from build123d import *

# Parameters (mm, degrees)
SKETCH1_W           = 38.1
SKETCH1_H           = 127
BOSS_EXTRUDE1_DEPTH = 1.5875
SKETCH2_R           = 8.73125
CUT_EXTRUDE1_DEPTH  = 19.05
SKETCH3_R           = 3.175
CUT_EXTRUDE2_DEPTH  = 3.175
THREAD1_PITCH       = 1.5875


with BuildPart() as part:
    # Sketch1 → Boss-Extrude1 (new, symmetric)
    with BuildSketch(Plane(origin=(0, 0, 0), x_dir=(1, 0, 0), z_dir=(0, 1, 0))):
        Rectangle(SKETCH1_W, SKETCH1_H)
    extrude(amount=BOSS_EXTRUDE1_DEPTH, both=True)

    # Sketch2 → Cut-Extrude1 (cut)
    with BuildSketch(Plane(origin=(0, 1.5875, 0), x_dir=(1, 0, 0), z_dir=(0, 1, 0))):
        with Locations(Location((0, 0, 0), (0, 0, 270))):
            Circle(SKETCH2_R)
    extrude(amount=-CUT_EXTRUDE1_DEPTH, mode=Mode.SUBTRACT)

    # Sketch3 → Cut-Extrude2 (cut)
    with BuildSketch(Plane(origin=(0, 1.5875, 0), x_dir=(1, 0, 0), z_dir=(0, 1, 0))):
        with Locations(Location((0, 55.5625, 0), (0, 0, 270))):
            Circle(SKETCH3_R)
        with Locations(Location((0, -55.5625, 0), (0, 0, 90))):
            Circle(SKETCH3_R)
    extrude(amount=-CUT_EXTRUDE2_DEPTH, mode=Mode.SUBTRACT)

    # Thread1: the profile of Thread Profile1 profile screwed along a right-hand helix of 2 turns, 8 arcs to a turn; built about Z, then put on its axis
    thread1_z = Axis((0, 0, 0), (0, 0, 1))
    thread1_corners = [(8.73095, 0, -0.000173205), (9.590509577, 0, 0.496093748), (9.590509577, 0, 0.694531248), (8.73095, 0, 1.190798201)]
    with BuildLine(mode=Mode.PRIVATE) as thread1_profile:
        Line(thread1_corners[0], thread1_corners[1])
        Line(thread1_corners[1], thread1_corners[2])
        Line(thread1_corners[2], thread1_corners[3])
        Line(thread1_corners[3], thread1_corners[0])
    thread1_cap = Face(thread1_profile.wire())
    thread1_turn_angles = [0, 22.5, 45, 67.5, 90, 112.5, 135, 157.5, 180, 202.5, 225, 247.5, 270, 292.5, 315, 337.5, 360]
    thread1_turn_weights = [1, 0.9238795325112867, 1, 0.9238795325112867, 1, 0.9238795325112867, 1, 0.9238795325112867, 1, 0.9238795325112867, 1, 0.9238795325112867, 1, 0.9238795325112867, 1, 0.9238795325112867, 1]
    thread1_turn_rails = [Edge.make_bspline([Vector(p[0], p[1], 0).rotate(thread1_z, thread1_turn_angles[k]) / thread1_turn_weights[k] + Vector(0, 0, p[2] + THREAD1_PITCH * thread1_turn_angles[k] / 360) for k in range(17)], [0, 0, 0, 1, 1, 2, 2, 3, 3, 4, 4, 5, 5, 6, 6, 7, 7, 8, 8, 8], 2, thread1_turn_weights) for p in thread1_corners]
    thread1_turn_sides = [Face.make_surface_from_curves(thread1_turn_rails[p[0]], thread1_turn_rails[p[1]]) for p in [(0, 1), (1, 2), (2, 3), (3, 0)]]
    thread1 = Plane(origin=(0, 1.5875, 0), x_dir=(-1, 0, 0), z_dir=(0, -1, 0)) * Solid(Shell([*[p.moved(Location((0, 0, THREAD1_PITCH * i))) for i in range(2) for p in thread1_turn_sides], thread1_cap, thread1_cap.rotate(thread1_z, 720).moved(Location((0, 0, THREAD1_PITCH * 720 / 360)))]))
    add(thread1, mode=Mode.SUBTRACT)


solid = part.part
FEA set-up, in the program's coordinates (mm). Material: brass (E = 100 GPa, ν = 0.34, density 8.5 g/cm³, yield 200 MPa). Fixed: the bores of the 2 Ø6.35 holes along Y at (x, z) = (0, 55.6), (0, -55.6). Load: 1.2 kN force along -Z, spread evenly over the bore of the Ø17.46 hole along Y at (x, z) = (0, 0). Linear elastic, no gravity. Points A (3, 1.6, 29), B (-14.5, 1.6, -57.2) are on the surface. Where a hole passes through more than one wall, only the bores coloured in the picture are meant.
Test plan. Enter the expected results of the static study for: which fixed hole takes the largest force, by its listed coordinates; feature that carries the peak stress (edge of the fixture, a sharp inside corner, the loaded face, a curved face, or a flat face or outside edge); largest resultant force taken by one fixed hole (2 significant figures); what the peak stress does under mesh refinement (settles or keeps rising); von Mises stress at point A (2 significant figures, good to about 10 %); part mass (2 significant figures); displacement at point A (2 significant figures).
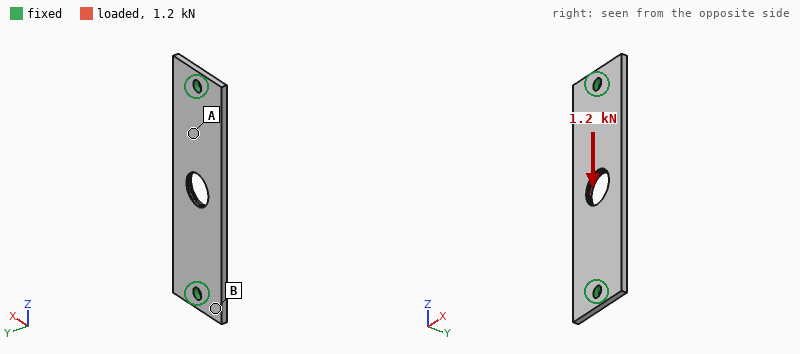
(0, 55.6)
a sharp inside corner
660 N
keeps rising
8.2 MPa
120 g
2.5 µm
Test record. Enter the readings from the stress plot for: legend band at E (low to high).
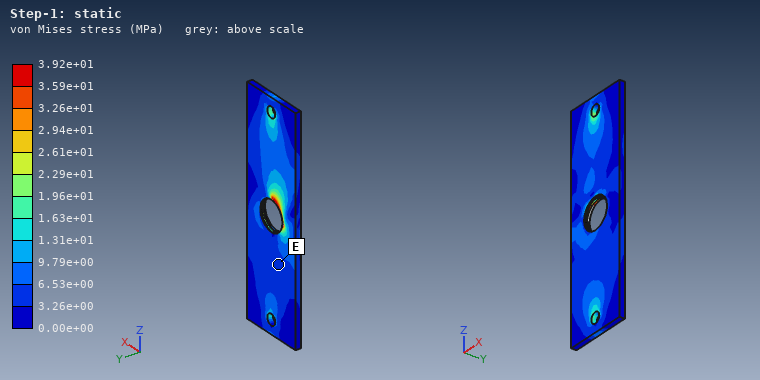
3.26e+00 to 6.53e+00 MPa
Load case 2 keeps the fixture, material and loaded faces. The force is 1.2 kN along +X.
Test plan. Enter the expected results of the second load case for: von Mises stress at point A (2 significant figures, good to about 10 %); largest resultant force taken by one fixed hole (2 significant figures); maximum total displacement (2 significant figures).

15 MPa
630 N
30 µm
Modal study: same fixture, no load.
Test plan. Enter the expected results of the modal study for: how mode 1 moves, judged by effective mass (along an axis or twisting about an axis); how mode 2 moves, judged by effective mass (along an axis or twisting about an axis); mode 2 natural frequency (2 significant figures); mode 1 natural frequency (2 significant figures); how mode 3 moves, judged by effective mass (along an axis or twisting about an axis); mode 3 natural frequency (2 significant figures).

along Y
twisting about Z
1600 Hz
910 Hz
twisting about X
2400 Hz
